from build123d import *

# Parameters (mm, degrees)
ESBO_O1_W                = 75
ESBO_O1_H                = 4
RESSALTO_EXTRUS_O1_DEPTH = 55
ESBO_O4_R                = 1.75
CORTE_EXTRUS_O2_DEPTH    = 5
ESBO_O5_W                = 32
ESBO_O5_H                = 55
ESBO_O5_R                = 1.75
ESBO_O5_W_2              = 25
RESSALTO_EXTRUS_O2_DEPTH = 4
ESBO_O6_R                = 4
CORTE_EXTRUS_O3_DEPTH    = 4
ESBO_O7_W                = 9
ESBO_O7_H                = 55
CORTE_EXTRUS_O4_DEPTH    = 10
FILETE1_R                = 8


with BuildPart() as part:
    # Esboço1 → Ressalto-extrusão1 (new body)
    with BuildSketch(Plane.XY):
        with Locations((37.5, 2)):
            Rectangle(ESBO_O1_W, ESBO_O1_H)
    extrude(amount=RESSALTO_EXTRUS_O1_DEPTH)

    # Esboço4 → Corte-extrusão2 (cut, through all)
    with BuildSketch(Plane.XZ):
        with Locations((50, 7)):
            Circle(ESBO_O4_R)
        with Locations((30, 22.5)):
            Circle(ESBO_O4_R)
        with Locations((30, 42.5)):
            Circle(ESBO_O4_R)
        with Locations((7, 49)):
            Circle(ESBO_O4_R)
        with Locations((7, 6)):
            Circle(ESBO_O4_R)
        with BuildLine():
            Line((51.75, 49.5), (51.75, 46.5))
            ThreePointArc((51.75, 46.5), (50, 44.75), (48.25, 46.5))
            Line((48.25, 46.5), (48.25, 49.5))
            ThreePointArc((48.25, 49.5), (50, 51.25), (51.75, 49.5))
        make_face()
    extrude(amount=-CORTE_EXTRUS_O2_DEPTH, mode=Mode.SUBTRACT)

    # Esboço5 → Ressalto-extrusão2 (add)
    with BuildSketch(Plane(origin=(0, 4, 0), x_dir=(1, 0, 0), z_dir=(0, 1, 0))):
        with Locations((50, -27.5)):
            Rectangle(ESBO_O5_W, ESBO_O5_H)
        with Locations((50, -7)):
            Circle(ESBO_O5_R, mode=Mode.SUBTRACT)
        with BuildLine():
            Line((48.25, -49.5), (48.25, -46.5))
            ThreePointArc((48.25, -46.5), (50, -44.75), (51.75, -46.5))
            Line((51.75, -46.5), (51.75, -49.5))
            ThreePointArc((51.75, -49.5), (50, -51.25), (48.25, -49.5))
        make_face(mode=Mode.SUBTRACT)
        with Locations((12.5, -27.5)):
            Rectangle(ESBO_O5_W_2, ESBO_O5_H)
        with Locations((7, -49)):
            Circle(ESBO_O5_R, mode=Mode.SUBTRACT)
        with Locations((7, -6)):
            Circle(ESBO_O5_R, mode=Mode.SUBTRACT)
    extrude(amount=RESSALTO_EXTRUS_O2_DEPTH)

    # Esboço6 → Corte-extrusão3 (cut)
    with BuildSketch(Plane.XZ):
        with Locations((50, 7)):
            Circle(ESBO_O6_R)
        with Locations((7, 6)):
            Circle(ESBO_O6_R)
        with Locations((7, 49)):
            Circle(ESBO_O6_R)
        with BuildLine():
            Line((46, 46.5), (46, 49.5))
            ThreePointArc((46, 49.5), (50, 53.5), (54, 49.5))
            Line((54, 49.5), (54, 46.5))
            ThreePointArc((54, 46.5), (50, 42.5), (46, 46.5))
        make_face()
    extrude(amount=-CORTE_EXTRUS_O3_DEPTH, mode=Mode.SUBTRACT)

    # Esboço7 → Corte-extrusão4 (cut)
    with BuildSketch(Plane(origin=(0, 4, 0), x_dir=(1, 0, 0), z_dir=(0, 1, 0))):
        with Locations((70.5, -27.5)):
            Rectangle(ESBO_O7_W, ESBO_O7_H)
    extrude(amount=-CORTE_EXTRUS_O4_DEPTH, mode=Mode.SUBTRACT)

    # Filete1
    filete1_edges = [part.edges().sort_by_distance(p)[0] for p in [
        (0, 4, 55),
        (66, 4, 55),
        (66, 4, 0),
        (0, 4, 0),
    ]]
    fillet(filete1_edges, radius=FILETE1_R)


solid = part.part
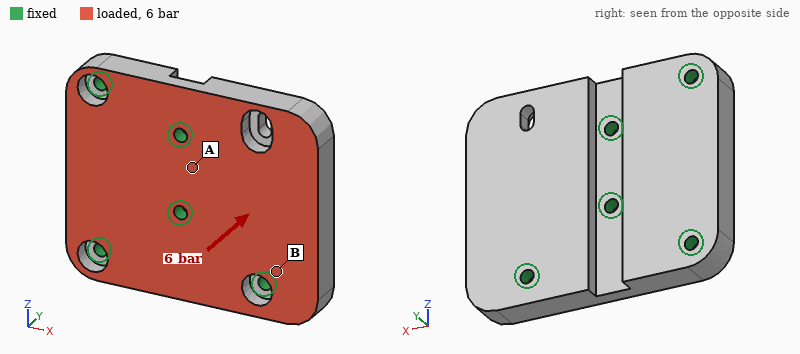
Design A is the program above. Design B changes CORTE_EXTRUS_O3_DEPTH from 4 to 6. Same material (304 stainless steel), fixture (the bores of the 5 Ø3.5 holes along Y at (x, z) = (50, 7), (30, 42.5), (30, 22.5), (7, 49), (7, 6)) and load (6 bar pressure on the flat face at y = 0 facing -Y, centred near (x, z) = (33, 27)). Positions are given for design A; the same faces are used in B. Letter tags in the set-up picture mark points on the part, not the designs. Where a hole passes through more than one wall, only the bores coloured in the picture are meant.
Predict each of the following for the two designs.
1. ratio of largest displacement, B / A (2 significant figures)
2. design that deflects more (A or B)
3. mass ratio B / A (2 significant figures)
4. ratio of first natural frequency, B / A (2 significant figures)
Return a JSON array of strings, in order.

["1.1", "B", "0.99", "0.94"]
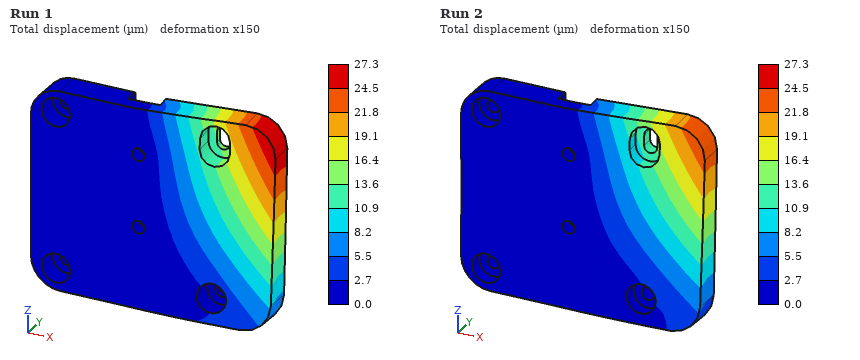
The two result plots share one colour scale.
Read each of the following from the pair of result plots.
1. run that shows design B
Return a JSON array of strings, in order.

["Run 1"]
